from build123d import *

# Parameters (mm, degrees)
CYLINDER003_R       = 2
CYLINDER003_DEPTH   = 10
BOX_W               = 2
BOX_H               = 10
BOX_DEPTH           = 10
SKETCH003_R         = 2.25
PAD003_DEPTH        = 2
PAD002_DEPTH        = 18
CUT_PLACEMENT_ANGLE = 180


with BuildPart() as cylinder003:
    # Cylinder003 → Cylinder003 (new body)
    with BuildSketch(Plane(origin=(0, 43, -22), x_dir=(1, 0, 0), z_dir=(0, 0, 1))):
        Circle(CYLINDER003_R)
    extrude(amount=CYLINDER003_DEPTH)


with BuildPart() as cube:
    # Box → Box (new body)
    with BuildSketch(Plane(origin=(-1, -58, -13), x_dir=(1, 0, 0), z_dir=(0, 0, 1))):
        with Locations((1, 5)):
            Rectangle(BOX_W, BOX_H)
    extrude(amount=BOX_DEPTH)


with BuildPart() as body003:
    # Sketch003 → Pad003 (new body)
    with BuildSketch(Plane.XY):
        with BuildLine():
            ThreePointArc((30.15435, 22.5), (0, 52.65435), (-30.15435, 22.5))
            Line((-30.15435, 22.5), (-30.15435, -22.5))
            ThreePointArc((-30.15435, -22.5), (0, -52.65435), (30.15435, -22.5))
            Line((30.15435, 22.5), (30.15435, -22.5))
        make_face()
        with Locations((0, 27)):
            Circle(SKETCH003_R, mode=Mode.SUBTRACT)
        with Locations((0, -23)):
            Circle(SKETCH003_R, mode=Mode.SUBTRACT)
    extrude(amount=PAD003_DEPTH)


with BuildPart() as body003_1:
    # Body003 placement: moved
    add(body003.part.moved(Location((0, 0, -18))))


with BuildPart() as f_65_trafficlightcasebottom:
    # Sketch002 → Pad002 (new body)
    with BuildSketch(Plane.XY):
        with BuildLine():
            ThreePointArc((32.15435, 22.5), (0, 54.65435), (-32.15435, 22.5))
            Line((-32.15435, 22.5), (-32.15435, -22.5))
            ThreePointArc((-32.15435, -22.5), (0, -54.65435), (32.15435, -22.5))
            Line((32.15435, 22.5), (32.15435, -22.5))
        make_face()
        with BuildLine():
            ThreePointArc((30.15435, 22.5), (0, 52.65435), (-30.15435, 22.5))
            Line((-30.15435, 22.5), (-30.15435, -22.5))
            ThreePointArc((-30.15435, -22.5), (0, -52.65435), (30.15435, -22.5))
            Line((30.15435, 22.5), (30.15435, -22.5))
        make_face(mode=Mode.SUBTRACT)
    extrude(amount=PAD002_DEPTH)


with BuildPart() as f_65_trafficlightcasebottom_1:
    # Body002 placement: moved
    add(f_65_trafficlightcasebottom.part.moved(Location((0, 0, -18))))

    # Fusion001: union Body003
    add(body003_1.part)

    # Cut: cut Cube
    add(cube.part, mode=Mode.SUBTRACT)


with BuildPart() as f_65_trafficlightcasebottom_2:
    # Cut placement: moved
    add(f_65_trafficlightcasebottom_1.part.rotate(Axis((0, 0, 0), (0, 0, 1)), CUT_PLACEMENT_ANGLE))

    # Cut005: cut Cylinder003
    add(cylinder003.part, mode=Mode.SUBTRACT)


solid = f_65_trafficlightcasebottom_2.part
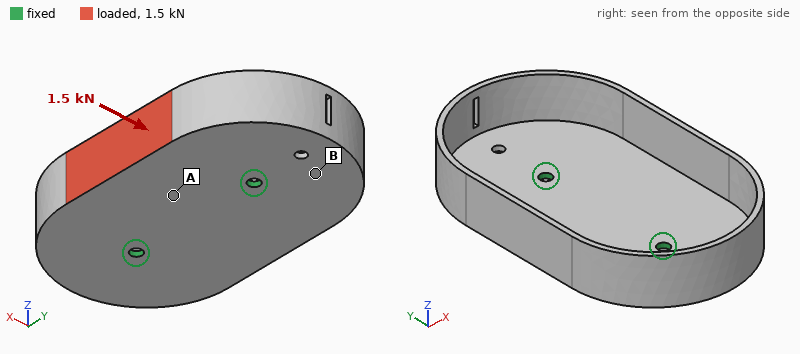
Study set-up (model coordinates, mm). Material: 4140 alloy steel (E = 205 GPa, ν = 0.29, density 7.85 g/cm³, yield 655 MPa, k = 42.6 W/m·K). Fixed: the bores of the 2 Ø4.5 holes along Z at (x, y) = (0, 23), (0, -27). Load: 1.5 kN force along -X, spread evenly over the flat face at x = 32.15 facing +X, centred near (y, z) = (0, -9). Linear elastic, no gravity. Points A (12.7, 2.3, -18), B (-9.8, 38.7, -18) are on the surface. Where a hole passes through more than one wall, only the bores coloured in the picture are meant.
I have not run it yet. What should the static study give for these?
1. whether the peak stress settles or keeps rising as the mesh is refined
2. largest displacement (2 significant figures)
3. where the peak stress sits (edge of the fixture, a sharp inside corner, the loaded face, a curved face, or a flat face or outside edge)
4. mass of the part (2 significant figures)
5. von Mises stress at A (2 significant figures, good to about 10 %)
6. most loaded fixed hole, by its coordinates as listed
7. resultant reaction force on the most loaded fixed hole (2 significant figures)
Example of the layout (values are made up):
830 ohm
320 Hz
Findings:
keeps rising
0.51 mm
edge of the fixture
170 g
80 MPa
(0, 23)
850 N
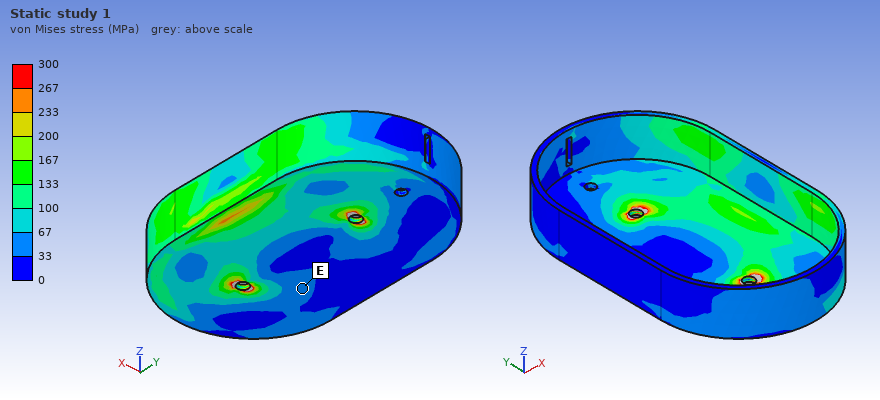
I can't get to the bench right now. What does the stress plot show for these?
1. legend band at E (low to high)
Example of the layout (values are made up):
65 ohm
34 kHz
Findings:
33 to 67 MPa
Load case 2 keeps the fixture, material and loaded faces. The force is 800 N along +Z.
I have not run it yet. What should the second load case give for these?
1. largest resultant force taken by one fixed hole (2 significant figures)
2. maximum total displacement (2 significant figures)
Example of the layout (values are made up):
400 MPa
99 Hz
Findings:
440 N
0.66 mm
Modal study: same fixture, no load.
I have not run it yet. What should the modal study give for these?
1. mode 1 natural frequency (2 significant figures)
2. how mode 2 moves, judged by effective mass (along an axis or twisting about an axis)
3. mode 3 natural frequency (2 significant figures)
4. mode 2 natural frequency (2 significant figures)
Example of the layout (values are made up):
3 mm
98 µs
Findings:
790 Hz
along Z
1500 Hz
1300 Hz
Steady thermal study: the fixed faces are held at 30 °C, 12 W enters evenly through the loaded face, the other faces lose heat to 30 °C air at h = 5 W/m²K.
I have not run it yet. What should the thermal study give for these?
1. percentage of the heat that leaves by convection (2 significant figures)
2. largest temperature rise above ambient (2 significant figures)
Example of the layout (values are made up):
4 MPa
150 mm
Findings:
20 %
75 K
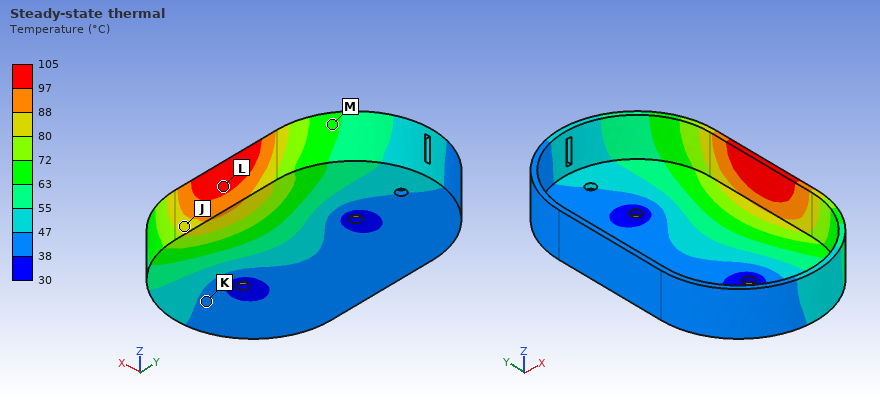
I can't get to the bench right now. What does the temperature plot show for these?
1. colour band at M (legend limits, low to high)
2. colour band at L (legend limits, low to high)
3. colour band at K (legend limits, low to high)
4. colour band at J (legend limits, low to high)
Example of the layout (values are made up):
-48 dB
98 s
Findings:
63 to 72 °C
97 to 105 °C
38 to 47 °C
80 to 88 °C
